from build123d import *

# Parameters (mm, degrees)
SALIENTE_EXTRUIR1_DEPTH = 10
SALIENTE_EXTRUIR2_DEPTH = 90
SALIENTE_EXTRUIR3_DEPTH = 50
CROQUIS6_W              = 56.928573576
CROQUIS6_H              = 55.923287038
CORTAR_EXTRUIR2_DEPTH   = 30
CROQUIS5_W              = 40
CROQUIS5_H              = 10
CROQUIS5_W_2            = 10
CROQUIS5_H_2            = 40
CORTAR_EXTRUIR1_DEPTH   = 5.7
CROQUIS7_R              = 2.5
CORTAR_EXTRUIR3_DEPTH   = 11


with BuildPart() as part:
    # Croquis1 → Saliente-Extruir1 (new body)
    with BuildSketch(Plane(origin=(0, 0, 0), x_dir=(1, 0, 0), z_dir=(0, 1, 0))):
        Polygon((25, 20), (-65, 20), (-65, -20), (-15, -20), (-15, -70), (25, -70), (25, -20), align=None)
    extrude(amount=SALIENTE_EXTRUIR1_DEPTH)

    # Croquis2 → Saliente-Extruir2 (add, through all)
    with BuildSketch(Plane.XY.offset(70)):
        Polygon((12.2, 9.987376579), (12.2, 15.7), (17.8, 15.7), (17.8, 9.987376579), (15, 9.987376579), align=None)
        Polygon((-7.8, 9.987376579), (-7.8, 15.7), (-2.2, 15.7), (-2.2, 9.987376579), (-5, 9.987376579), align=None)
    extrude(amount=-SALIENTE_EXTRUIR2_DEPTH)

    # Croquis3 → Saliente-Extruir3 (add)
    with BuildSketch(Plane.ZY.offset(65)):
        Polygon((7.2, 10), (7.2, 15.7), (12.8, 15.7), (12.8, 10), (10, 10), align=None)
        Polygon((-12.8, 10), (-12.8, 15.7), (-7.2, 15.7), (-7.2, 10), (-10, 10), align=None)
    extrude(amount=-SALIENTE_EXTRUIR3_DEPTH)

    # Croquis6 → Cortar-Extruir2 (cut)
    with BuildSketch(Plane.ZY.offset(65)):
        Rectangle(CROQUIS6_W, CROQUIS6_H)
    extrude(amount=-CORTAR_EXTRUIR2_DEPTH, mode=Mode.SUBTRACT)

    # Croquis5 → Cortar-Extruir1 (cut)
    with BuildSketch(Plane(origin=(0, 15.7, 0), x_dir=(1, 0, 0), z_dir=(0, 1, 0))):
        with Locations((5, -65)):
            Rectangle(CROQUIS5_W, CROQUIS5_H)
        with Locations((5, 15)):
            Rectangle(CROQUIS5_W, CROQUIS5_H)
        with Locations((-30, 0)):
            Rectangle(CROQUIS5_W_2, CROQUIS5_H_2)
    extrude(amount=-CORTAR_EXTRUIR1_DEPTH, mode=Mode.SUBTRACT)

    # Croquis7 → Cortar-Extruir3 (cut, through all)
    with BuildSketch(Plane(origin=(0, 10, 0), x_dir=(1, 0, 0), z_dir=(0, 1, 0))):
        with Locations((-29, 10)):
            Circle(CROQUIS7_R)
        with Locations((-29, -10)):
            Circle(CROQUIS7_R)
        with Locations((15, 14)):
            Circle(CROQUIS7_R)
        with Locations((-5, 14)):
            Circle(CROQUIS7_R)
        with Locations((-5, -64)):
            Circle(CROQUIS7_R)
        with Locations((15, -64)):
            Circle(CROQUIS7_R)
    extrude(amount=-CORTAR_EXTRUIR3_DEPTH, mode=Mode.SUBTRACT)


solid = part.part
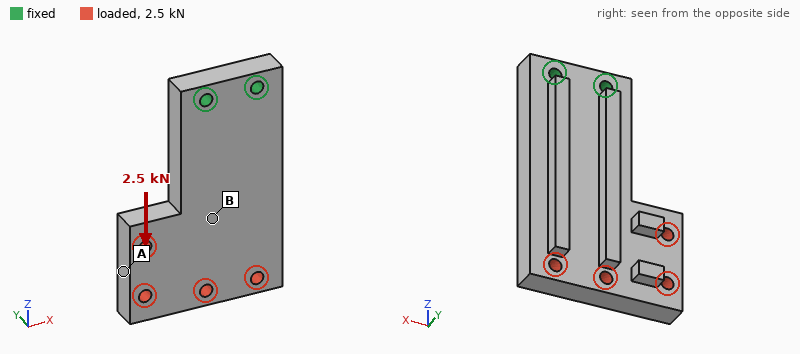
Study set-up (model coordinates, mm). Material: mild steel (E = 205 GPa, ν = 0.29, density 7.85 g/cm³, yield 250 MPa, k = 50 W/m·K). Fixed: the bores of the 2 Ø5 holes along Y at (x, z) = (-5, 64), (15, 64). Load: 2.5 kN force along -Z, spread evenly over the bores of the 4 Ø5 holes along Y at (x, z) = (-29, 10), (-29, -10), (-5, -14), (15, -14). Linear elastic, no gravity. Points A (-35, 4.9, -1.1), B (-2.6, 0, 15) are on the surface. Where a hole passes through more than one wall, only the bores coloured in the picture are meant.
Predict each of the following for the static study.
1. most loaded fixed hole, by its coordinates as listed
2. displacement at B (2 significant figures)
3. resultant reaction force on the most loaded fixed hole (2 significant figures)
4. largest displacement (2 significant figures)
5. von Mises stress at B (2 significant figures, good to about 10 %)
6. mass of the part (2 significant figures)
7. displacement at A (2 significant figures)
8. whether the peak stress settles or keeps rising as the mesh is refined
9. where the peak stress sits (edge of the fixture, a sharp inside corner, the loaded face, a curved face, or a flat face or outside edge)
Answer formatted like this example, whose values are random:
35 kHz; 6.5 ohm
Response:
(-5, 64); 6.7 µm; 3.1 kN; 20 µm; 8.7 MPa; 380 g; 16 µm; keeps rising; edge of the fixture
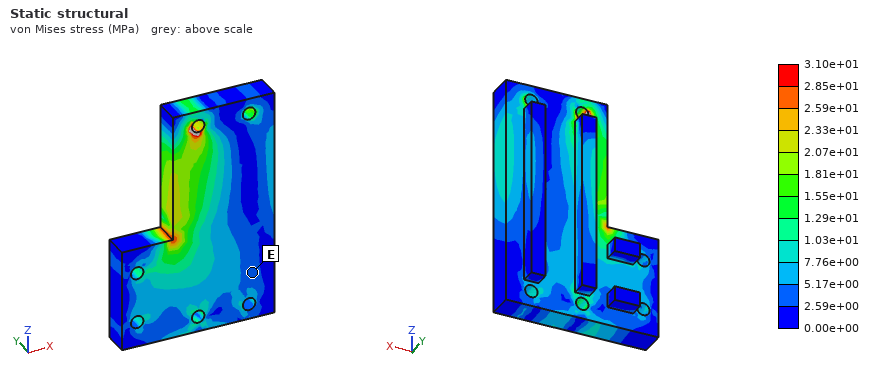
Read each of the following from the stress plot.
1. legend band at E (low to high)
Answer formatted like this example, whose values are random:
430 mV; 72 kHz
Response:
2.59e+00 to 5.17e+00 MPa
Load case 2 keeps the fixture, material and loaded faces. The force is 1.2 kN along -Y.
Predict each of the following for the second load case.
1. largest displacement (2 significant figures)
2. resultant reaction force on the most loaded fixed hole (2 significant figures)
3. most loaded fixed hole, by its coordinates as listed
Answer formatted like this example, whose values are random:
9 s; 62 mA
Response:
0.23 mm; 1.3 kN; (-5, 64)
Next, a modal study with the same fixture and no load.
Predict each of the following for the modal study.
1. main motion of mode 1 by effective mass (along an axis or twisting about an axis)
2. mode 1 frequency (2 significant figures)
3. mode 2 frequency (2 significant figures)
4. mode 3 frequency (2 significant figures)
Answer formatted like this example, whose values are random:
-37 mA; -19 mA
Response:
along Y; 1100 Hz; 2900 Hz; 2900 Hz
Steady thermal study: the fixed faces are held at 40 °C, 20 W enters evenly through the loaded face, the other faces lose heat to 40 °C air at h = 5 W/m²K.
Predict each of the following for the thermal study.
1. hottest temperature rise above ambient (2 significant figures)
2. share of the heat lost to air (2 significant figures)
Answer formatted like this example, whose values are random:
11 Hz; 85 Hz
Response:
62 K; 12 %
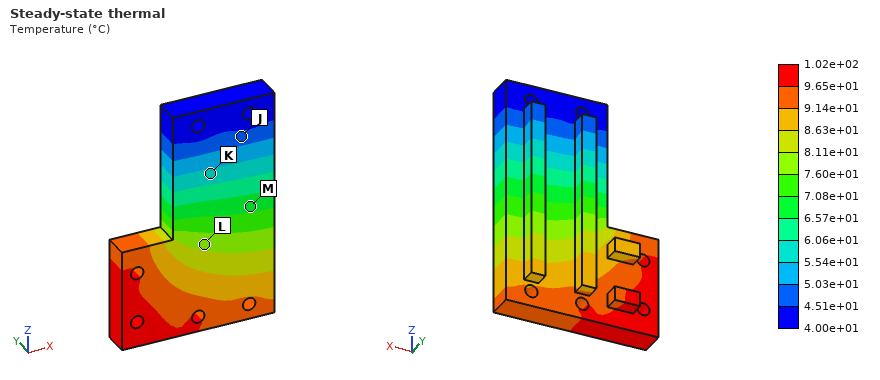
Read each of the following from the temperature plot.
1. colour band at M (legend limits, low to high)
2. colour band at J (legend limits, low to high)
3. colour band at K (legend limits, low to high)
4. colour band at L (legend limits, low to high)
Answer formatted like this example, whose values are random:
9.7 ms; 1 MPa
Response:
6.57e+01 to 7.08e+01 °C; 4.51e+01 to 5.03e+01 °C; 5.54e+01 to 6.06e+01 °C; 7.60e+01 to 8.11e+01 °C
